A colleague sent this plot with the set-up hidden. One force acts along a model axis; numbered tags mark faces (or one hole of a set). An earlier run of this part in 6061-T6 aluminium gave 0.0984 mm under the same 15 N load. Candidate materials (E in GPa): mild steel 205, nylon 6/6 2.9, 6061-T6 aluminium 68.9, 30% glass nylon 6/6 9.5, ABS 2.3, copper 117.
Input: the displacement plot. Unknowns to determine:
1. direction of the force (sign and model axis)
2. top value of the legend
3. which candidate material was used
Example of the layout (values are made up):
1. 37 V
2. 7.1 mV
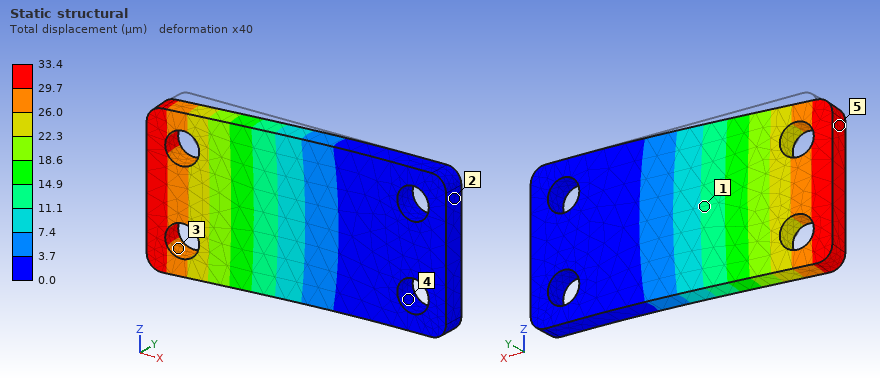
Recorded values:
1. -Y
2. 33.4 µm
3. mild steel
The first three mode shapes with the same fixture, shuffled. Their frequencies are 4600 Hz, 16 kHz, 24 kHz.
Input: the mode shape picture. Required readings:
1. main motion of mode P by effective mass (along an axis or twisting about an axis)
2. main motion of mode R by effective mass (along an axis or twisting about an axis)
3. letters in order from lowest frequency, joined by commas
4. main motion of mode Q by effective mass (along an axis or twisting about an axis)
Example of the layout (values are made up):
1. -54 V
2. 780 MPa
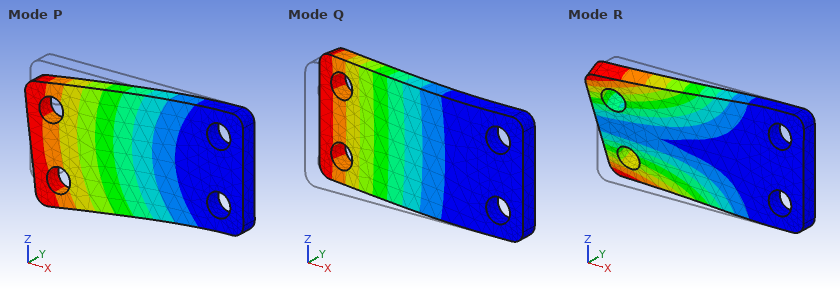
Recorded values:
1. along Z
2. twisting about X
3. Q, R, P
4. along Y
